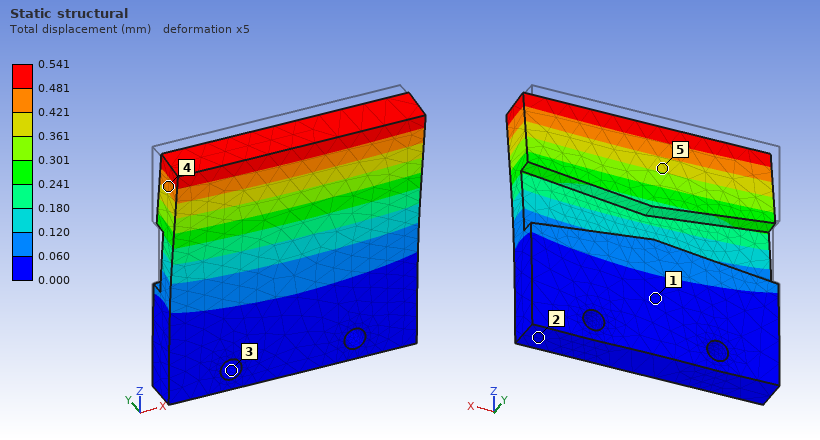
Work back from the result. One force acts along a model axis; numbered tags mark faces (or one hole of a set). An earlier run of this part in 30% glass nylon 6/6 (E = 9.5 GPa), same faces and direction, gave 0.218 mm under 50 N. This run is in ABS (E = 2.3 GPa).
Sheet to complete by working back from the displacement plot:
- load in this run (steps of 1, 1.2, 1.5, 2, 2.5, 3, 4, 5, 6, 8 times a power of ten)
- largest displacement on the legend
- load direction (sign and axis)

30 N
0.541 mm
-Y
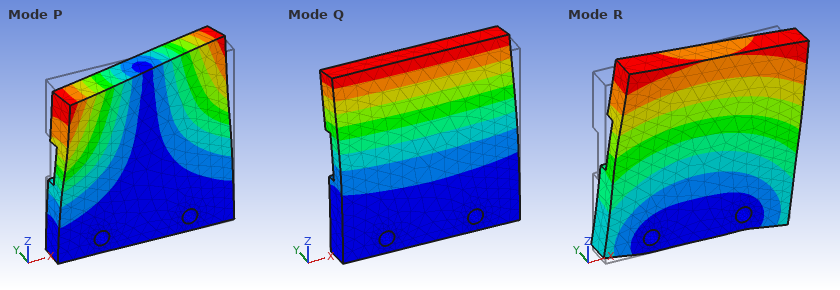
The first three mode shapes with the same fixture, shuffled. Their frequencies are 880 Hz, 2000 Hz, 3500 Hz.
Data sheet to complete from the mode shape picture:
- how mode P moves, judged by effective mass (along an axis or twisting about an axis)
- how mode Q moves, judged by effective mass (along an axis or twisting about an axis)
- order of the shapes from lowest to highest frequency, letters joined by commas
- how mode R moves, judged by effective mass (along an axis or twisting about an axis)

twisting about Z
along Y
Q, P, R
along X
